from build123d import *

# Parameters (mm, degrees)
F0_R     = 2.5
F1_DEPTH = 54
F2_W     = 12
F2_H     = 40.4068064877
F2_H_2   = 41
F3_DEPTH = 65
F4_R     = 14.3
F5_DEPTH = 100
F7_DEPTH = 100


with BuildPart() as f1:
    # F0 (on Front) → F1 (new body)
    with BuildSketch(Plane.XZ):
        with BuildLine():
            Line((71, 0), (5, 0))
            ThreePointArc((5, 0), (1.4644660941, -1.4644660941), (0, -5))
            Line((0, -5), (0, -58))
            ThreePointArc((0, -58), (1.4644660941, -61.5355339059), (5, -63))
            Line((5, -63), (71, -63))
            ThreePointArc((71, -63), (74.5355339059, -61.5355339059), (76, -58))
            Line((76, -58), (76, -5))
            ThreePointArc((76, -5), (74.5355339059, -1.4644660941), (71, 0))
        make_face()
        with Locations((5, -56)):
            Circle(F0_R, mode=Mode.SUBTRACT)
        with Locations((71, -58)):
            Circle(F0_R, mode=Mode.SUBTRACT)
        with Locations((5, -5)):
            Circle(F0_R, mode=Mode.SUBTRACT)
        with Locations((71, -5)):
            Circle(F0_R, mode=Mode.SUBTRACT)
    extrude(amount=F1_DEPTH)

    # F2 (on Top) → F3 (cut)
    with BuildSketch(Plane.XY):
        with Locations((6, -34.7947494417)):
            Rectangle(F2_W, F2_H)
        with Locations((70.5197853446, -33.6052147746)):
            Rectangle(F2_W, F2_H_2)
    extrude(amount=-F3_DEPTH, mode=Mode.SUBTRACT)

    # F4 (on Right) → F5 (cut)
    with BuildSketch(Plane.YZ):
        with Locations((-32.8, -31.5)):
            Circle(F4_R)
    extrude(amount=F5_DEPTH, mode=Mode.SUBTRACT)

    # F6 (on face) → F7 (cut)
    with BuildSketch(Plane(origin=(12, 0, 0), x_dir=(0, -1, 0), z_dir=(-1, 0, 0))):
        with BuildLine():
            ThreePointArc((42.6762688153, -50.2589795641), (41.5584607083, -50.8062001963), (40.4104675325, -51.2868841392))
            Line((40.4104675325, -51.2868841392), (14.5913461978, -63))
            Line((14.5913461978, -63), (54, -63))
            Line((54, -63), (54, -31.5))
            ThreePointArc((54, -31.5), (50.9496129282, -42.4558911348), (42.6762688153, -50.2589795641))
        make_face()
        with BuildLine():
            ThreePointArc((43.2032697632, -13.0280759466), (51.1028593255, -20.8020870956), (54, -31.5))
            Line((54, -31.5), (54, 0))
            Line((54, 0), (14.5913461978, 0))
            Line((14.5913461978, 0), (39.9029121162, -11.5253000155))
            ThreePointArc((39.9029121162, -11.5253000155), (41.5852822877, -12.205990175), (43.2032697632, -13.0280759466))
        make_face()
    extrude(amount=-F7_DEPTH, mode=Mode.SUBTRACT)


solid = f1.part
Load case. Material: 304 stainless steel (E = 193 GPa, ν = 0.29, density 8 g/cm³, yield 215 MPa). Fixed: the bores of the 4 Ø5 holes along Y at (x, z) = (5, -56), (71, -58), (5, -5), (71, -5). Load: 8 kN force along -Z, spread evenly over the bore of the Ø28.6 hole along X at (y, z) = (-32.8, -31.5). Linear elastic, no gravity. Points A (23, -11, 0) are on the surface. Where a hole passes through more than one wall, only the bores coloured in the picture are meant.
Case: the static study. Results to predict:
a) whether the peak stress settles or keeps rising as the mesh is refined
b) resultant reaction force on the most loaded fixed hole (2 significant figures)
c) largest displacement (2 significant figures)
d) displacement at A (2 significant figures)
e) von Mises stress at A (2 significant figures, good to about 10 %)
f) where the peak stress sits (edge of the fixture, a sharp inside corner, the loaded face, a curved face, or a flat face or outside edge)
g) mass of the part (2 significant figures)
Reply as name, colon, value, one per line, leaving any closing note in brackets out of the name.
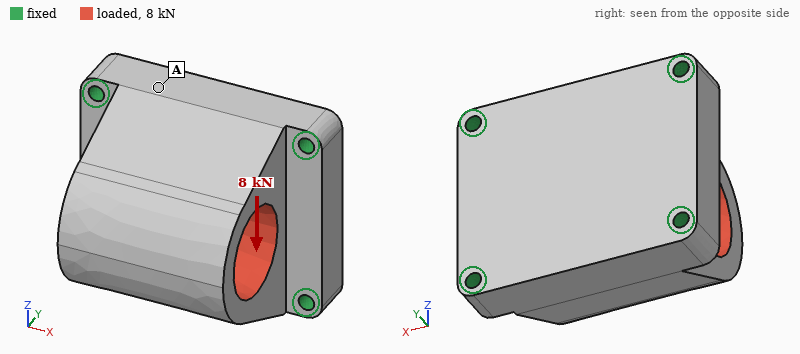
whether the peak stress settles or keeps rising as the mesh is refined: keeps rising
resultant reaction force on the most loaded fixed hole: 3.2 kN
largest displacement: 10 µm
displacement at A: 3.3 µm
von Mises stress at A: 6.9 MPa
where the peak stress sits: edge of the fixture
mass of the part: 990 g
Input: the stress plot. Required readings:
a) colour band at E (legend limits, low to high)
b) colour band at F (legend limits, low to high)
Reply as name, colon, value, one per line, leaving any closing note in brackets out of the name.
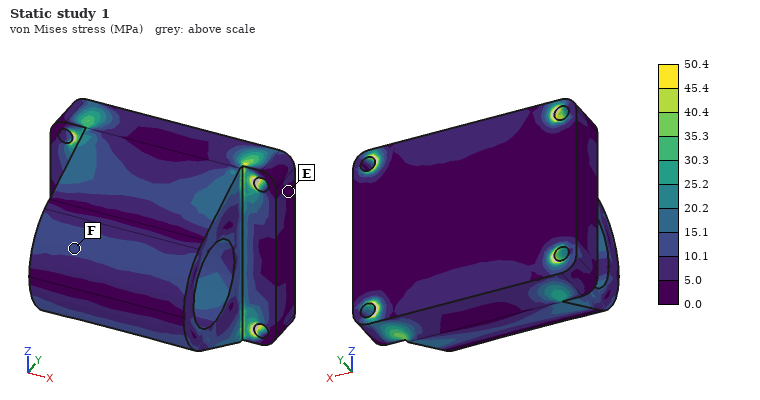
colour band at E: 0.0 to 5.0 MPa
colour band at F: 10.1 to 15.1 MPa
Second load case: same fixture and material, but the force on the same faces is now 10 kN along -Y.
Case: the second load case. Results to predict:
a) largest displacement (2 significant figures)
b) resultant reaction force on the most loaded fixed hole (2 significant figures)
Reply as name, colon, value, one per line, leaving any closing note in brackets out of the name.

largest displacement: 4.7 µm
resultant reaction force on the most loaded fixed hole: 2.7 kN
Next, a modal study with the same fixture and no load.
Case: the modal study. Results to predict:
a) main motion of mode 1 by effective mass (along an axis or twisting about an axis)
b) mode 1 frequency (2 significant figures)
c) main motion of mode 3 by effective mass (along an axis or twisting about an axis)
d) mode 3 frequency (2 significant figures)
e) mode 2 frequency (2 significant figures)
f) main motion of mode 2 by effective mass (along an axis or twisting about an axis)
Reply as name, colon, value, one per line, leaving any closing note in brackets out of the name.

main motion of mode 1 by effective mass: along Z
mode 1 frequency: 8000 Hz
main motion of mode 3 by effective mass: along X
mode 3 frequency: 10 kHz
mode 2 frequency: 9700 Hz
main motion of mode 2 by effective mass: along Y
